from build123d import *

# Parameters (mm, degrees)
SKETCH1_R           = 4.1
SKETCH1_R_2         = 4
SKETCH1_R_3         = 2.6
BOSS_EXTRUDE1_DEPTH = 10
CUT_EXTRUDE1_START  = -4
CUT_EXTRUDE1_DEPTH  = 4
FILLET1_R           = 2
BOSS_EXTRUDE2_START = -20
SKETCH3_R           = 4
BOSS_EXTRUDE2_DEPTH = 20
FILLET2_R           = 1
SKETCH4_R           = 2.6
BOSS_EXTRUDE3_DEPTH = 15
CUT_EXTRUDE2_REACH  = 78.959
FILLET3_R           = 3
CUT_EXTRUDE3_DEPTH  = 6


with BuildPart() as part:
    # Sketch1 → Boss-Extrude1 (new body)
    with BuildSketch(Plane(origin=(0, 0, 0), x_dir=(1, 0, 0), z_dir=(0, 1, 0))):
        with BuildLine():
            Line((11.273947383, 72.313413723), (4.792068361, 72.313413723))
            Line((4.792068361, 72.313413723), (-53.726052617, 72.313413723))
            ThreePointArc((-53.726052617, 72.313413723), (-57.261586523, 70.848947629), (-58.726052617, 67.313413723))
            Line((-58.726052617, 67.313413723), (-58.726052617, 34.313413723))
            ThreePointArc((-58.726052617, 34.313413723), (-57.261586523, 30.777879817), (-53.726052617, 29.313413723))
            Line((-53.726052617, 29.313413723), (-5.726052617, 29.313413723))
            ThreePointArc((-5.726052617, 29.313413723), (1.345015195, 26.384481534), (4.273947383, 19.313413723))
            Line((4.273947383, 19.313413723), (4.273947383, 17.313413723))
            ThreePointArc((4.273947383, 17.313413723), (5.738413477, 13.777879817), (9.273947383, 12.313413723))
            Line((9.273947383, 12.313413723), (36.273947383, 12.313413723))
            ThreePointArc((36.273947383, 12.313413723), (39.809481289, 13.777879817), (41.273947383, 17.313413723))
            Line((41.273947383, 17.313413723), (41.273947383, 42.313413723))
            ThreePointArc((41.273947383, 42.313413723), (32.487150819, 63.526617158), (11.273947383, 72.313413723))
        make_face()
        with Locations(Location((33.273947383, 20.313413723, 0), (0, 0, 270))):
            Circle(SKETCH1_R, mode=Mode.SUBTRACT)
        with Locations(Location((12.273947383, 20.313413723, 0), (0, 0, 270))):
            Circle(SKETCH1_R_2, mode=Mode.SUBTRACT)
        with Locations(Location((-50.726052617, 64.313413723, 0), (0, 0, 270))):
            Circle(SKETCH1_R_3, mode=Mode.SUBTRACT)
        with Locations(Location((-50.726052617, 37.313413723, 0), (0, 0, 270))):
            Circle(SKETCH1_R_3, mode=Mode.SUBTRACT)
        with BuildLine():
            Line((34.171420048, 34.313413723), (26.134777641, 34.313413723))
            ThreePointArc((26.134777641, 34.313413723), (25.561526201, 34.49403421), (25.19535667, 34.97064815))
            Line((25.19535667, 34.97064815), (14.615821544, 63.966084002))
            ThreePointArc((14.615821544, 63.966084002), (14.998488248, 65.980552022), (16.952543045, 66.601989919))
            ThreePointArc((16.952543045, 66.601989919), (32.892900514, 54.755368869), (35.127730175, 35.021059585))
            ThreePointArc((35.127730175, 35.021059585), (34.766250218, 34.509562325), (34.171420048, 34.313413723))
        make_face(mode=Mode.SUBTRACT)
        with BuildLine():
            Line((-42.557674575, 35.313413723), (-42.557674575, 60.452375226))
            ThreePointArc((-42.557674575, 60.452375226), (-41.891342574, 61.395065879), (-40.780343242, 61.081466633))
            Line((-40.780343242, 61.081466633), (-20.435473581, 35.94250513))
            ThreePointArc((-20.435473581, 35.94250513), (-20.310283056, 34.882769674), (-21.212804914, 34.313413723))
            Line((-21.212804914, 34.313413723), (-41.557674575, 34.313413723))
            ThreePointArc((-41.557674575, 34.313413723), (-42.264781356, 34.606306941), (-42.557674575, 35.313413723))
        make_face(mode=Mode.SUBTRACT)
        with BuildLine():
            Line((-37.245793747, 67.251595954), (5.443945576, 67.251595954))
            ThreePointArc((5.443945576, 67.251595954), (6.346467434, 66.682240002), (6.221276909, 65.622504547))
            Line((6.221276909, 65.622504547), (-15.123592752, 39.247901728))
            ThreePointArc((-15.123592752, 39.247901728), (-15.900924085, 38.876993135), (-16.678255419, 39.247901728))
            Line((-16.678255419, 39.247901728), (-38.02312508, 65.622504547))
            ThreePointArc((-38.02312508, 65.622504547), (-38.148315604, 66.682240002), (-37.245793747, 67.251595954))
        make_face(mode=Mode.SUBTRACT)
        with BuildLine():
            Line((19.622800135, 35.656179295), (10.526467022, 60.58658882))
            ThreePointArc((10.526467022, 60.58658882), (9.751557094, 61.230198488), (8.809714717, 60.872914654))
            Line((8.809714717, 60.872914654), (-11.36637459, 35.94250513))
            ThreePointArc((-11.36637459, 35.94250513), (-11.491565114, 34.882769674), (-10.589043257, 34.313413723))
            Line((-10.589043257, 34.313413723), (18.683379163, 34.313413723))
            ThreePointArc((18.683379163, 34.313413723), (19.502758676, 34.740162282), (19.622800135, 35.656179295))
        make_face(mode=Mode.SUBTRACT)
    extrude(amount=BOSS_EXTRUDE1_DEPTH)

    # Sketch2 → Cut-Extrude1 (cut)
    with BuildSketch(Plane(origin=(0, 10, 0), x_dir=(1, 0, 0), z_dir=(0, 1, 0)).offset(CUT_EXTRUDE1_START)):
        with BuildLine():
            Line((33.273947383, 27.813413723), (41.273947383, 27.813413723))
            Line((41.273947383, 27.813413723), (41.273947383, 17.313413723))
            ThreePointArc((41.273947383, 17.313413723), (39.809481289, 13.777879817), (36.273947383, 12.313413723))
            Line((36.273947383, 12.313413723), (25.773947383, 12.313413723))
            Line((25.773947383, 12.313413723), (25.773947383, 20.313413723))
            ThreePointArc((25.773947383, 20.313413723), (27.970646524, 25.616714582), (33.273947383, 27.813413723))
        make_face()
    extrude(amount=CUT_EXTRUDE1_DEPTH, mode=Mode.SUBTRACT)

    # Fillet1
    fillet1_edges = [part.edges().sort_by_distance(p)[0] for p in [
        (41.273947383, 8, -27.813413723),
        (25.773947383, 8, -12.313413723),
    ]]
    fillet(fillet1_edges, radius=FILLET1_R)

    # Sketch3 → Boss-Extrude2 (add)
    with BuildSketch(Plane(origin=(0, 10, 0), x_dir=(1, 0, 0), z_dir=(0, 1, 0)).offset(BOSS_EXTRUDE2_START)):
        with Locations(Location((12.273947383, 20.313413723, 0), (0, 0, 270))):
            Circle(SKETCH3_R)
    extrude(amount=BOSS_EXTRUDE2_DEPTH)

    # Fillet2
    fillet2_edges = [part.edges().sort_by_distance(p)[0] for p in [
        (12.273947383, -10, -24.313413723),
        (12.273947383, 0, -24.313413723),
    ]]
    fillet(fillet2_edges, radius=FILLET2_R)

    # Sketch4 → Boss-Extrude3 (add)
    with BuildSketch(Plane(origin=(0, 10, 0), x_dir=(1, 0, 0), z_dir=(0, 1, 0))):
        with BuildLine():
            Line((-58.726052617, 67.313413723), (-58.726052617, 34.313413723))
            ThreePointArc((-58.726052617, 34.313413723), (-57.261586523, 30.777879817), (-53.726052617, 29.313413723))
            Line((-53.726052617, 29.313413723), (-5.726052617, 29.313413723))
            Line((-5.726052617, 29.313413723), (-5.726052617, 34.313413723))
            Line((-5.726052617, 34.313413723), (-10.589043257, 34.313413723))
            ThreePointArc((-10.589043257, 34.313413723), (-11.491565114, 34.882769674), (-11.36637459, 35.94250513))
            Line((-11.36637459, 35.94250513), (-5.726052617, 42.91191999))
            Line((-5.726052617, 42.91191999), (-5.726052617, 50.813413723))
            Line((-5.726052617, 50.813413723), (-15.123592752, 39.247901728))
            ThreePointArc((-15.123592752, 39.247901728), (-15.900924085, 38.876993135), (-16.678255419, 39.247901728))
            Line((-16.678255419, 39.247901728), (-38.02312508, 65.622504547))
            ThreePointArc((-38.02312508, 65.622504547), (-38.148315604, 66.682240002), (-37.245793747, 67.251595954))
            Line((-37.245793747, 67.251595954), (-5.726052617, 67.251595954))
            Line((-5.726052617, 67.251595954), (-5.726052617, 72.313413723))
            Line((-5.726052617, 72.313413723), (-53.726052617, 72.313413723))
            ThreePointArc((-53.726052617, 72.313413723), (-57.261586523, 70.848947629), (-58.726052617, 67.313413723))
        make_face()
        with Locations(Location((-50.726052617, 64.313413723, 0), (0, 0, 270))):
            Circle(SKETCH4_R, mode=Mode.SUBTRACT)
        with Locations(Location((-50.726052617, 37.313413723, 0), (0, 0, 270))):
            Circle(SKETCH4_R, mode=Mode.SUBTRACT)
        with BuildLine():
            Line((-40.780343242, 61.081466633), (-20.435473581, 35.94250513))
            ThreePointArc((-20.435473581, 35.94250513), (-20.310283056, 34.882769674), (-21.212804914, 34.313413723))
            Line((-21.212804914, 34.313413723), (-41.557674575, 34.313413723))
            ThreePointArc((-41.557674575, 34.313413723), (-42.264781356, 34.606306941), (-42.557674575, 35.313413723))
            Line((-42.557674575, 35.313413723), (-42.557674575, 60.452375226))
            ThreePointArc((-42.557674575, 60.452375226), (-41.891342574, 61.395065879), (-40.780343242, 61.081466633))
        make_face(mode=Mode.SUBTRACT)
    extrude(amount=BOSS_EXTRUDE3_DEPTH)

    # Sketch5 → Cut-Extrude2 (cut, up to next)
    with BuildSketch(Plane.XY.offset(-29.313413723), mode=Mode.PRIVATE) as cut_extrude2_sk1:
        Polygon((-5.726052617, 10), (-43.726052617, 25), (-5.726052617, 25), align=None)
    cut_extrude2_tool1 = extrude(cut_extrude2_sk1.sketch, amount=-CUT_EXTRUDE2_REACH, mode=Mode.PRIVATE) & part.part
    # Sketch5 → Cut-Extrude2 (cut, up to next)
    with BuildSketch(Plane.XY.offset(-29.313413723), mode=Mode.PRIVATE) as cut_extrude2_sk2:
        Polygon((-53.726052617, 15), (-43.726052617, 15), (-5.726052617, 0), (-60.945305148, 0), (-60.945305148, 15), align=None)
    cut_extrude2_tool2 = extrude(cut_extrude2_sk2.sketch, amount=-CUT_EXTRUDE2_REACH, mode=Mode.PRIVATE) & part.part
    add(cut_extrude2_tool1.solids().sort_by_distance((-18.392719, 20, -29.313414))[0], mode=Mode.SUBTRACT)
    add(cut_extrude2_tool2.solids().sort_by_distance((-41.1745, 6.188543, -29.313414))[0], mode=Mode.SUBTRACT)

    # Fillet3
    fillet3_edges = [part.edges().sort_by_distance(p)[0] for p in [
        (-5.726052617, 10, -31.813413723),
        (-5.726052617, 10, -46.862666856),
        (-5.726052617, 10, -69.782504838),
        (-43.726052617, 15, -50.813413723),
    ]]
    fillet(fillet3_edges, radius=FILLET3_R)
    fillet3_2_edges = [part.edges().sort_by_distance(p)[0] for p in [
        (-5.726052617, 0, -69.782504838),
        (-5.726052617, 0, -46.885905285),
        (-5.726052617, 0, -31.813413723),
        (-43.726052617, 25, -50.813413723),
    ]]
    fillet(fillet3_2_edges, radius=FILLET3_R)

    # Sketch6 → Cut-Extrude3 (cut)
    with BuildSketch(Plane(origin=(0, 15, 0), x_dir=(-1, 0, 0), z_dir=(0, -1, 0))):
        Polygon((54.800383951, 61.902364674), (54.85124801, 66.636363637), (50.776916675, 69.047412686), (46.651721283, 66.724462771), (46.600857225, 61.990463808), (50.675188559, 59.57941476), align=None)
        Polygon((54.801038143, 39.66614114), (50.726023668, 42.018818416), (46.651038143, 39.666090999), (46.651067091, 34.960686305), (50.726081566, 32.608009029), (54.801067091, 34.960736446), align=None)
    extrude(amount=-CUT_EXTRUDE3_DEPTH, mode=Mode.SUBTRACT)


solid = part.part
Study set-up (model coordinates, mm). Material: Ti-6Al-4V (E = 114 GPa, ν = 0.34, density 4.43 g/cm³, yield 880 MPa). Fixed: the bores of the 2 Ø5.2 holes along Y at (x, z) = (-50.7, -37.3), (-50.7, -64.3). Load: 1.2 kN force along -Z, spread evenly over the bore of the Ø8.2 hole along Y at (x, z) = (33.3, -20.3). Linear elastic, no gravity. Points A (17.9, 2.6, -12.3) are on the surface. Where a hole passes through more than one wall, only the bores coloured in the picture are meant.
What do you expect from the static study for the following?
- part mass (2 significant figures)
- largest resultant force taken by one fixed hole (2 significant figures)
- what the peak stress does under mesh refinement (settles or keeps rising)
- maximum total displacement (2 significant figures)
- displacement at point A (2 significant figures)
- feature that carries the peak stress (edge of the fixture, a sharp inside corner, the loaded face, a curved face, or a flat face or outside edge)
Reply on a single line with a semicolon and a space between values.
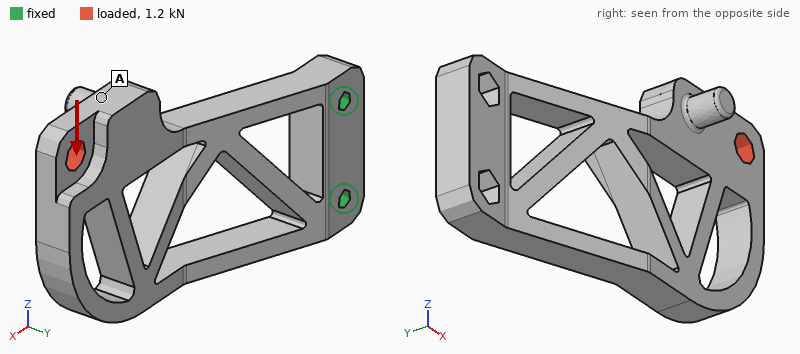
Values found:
120 g; 3.3 kN; keeps rising; 0.27 mm; 0.21 mm; edge of the fixture
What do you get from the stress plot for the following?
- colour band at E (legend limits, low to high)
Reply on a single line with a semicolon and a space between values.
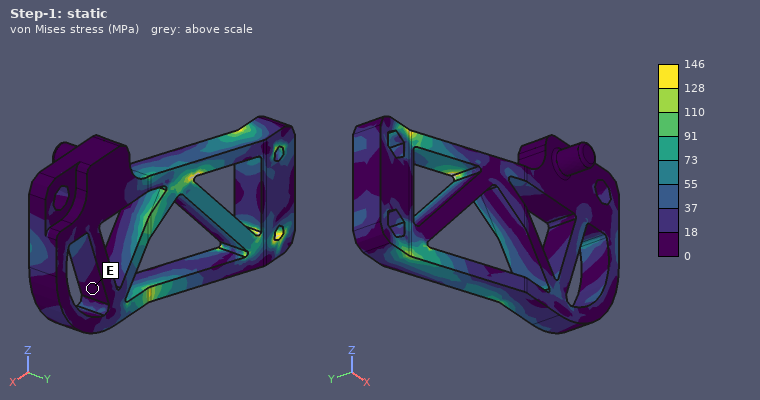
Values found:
0 to 18 MPa
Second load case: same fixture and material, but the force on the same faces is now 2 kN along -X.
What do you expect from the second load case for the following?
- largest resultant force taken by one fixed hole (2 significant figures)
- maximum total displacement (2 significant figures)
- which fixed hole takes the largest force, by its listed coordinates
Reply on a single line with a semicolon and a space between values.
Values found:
2.9 kN; 1.2 mm; (-50.7, -37.3)
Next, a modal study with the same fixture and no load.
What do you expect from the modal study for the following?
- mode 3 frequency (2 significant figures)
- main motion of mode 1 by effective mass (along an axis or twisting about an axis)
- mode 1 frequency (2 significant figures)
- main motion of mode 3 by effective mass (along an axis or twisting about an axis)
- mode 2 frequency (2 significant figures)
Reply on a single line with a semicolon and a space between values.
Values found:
2300 Hz; along Y; 500 Hz; along Z; 1500 Hz
